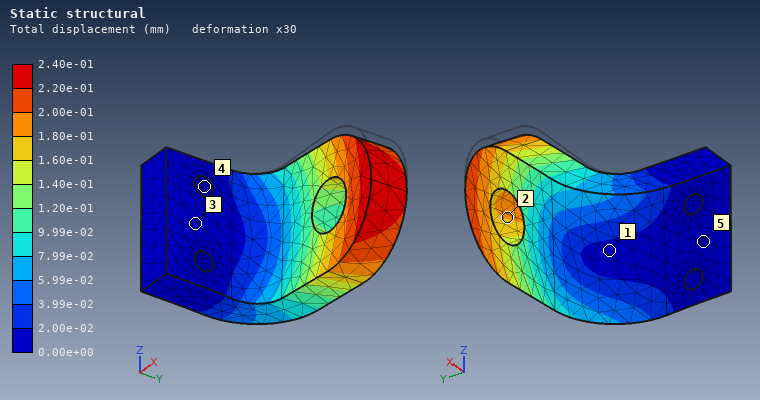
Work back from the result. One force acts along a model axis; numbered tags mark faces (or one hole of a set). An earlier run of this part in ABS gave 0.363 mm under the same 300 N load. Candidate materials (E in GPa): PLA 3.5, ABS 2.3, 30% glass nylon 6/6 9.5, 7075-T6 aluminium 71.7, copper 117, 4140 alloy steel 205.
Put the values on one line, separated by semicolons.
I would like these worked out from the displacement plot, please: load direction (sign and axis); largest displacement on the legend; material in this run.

-Z; 2.40e-01 mm; PLA
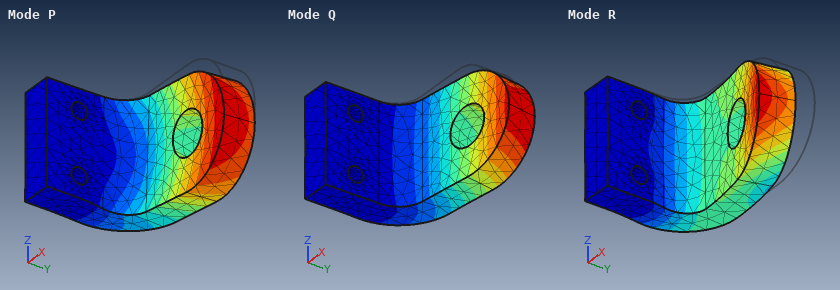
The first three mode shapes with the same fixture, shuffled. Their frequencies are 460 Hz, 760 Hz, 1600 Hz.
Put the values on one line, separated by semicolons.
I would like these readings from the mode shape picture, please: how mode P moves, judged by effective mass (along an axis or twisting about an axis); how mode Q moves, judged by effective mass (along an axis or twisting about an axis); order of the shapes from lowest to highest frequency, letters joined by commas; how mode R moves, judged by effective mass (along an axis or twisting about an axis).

along Z; along Y; Q, P, R; along X
